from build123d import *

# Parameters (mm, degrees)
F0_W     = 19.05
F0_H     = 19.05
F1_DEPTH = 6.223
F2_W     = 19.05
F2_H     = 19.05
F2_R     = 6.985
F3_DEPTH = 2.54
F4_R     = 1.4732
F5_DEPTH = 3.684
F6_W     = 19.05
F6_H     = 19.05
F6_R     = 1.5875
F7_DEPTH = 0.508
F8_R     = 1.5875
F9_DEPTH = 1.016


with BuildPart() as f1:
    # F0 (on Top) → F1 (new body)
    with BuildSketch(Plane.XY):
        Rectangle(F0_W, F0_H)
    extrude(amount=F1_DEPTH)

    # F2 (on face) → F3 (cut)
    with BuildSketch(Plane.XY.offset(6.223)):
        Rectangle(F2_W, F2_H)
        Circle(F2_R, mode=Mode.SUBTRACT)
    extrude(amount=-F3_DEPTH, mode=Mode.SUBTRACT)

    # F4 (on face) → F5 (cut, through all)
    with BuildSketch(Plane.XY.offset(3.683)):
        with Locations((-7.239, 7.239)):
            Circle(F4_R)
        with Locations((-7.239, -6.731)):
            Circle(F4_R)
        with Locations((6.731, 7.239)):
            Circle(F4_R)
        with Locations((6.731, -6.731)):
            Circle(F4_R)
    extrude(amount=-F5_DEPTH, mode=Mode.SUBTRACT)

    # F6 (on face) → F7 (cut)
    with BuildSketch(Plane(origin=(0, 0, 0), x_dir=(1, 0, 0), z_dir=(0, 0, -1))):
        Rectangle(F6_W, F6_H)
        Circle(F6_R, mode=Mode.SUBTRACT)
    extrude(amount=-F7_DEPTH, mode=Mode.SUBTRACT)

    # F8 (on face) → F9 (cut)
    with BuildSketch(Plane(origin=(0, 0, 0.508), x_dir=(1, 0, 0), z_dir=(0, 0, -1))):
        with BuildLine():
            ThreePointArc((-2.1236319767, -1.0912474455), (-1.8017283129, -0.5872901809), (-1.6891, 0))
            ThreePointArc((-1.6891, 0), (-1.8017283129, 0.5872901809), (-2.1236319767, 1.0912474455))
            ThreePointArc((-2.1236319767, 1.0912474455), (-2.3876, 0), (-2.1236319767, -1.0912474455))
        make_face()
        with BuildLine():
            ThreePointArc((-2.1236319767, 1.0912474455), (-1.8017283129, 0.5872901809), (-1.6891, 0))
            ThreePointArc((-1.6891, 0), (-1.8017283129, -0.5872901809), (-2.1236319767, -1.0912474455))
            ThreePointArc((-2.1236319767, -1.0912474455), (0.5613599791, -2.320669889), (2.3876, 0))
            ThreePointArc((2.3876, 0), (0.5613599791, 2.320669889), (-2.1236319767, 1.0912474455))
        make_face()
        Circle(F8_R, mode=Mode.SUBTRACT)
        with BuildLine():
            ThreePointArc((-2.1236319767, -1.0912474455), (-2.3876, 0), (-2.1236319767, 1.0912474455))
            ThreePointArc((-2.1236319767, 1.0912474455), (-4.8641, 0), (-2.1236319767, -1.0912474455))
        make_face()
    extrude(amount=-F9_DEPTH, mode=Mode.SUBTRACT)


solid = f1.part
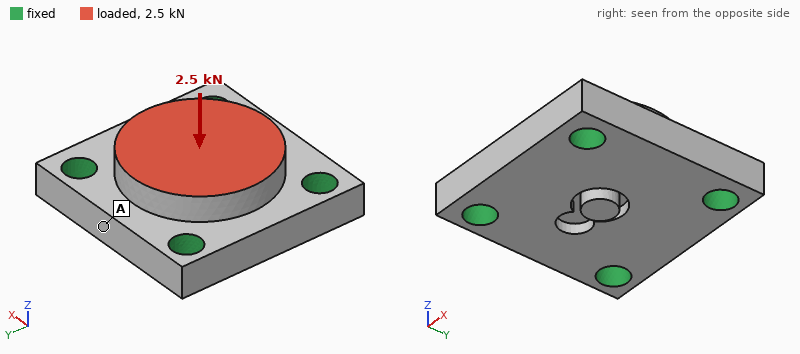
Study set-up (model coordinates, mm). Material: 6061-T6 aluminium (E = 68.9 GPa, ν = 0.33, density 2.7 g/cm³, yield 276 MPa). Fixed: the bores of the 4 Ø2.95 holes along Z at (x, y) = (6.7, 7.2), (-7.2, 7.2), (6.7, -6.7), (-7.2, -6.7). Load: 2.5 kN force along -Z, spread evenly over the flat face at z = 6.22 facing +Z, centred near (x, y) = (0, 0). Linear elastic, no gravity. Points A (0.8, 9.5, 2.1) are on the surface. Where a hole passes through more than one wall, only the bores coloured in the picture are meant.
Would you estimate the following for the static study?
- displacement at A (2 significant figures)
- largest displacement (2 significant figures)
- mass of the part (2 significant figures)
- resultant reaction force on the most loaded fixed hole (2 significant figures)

3.7 µm
8.7 µm
3.9 g
720 N
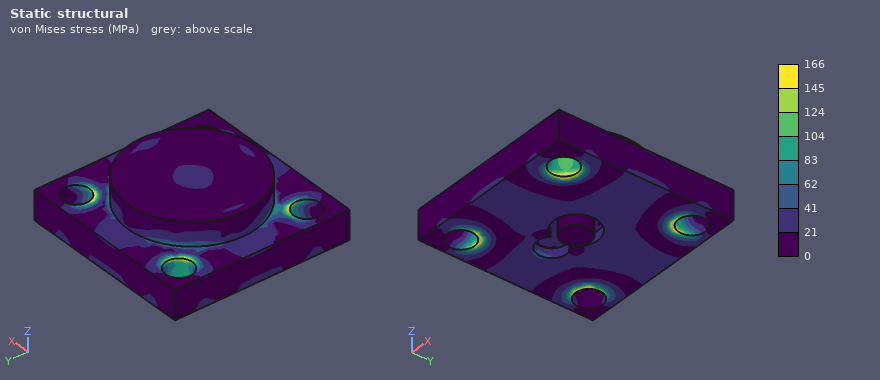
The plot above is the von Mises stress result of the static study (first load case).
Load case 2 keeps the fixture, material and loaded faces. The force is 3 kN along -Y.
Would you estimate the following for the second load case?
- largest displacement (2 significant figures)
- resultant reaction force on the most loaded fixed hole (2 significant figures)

11 µm
1.0 kN
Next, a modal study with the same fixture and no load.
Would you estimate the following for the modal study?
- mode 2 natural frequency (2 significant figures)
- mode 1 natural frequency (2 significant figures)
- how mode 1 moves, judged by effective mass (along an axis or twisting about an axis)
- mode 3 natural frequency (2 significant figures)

79 kHz
58 kHz
along Z
79 kHz
